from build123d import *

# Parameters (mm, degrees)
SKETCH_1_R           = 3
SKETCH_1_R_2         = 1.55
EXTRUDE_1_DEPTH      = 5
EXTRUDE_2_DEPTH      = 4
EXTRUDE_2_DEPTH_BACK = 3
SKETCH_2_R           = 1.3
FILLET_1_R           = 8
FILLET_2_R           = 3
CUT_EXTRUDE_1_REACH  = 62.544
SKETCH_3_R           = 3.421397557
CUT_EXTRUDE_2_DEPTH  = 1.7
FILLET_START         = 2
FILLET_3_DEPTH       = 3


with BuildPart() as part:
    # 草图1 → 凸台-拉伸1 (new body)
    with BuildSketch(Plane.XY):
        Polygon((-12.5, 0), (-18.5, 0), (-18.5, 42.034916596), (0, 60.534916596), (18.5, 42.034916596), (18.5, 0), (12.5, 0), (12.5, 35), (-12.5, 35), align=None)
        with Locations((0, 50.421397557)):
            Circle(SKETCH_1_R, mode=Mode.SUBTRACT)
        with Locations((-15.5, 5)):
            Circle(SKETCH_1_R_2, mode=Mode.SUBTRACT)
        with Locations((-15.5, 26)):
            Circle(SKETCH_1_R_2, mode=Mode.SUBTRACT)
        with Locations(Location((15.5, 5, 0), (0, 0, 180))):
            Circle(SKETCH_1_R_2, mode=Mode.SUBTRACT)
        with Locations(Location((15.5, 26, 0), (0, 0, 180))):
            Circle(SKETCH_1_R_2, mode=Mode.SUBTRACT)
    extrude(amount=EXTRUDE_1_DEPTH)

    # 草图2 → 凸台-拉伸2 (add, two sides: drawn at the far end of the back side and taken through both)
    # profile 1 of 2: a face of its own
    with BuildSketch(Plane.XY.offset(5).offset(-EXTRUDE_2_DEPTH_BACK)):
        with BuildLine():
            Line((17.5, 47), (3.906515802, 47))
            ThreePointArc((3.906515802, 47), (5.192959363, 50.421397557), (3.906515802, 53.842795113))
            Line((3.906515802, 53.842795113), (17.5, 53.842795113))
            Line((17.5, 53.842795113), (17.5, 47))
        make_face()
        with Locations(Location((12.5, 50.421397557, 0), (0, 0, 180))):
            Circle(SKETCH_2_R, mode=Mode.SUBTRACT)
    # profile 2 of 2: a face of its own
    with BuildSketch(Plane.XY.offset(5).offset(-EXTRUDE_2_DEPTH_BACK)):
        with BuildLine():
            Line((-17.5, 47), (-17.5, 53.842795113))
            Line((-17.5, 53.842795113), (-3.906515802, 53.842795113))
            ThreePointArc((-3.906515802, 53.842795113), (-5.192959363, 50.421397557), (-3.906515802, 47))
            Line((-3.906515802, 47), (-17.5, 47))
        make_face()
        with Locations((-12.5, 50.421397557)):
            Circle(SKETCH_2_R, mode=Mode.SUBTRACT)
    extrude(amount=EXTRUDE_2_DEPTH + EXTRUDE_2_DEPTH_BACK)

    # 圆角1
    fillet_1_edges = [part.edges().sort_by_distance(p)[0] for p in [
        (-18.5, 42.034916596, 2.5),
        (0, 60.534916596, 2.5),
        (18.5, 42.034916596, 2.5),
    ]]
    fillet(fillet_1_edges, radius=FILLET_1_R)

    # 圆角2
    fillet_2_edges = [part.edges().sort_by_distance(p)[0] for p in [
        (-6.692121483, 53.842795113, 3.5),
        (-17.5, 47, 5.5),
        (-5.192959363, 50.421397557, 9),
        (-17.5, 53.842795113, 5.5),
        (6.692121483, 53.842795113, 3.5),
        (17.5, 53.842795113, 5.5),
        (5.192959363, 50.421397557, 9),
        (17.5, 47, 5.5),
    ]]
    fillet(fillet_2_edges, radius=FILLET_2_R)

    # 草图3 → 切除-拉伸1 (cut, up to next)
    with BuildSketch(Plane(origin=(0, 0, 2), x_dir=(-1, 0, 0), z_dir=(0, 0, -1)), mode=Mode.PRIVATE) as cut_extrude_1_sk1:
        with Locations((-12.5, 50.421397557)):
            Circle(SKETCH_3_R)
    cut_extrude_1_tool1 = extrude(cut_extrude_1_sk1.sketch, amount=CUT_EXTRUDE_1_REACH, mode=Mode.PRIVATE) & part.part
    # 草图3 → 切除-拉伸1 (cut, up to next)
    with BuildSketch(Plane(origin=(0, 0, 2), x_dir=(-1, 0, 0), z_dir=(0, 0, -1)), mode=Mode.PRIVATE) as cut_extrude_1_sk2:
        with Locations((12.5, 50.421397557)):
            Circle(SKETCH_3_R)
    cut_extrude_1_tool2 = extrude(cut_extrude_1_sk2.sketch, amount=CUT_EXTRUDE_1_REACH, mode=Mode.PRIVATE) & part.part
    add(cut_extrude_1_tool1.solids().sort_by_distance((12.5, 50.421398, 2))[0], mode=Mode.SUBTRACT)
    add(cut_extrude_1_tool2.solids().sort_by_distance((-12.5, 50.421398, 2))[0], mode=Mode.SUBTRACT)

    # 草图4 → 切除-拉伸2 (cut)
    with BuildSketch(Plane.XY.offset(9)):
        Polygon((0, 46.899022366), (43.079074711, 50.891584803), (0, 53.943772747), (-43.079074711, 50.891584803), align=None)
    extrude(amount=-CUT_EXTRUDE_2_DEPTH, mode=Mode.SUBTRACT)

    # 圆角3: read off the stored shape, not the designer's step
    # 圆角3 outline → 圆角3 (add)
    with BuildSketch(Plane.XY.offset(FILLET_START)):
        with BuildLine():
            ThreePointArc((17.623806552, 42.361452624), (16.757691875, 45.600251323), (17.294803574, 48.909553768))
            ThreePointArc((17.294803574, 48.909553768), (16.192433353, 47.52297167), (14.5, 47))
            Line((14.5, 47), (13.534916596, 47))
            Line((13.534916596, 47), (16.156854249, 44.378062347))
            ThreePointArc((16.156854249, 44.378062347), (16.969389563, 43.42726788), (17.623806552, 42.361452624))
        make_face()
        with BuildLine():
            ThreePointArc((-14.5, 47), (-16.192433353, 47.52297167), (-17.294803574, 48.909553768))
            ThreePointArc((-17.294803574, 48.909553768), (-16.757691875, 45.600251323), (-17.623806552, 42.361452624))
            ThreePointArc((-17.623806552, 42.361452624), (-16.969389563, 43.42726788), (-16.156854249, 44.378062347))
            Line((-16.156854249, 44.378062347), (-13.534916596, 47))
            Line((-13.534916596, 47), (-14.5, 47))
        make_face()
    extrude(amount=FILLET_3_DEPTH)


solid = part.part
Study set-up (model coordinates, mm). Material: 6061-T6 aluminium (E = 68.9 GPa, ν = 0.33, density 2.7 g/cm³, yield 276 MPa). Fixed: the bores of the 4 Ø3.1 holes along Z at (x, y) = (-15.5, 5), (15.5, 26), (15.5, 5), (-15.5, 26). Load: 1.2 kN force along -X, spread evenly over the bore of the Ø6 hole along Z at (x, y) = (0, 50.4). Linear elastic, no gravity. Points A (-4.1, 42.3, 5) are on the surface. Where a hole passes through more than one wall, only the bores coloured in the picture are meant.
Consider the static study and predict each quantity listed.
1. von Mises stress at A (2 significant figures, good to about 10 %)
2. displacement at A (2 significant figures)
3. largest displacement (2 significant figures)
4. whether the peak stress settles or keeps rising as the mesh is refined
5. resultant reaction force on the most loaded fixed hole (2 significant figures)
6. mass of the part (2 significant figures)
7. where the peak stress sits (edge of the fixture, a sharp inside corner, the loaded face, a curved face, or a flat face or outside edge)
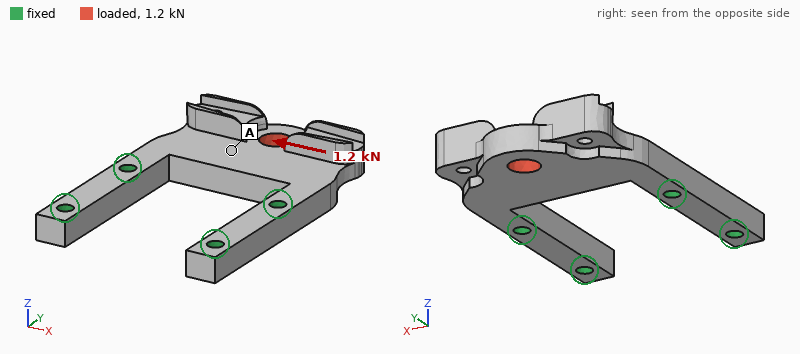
17 MPa
26 µm
34 µm
keeps rising
940 N
15 g
edge of the fixture
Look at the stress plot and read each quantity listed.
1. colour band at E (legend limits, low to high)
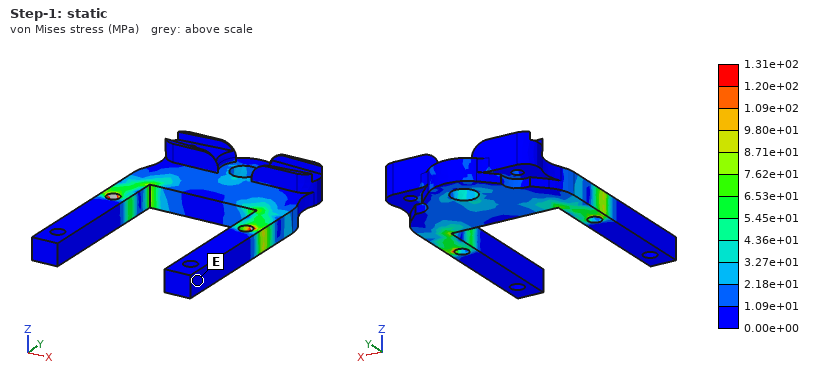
0.00e+00 to 1.09e+01 MPa
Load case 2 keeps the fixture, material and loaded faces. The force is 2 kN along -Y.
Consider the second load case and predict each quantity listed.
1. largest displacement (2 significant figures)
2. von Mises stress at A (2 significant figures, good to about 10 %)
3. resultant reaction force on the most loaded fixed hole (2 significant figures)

18 µm
16 MPa
1.0 kN
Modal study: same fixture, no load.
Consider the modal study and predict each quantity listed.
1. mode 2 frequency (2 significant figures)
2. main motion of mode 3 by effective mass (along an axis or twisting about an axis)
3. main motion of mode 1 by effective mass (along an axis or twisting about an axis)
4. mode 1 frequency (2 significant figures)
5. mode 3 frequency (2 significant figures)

9200 Hz
along X
along Z
3000 Hz
11 kHz
